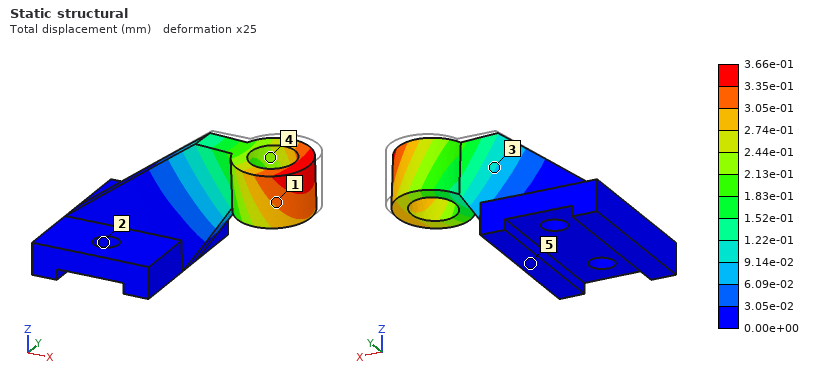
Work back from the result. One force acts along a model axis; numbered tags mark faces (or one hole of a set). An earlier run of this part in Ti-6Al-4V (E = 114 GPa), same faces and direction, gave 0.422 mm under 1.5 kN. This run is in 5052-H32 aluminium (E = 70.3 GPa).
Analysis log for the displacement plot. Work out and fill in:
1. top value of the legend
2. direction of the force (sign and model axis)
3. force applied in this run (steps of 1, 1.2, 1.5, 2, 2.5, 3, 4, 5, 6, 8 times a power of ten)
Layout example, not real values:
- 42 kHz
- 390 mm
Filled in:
- 3.66e-01 mm
- -Y
- 800 N
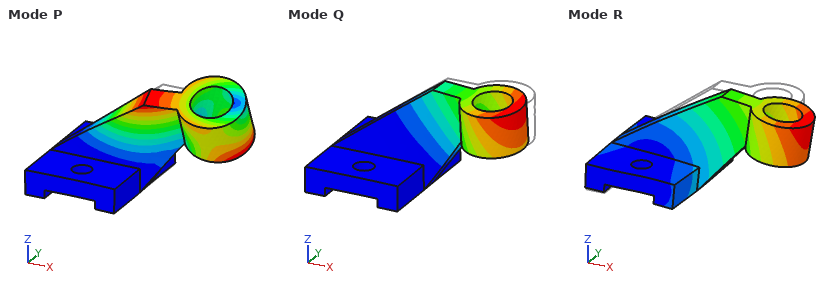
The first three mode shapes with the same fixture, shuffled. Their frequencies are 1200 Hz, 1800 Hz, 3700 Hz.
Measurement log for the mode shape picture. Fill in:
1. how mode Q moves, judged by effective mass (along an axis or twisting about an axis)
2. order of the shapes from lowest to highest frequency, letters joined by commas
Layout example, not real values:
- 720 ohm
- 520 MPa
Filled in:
- along Y
- Q, R, P
